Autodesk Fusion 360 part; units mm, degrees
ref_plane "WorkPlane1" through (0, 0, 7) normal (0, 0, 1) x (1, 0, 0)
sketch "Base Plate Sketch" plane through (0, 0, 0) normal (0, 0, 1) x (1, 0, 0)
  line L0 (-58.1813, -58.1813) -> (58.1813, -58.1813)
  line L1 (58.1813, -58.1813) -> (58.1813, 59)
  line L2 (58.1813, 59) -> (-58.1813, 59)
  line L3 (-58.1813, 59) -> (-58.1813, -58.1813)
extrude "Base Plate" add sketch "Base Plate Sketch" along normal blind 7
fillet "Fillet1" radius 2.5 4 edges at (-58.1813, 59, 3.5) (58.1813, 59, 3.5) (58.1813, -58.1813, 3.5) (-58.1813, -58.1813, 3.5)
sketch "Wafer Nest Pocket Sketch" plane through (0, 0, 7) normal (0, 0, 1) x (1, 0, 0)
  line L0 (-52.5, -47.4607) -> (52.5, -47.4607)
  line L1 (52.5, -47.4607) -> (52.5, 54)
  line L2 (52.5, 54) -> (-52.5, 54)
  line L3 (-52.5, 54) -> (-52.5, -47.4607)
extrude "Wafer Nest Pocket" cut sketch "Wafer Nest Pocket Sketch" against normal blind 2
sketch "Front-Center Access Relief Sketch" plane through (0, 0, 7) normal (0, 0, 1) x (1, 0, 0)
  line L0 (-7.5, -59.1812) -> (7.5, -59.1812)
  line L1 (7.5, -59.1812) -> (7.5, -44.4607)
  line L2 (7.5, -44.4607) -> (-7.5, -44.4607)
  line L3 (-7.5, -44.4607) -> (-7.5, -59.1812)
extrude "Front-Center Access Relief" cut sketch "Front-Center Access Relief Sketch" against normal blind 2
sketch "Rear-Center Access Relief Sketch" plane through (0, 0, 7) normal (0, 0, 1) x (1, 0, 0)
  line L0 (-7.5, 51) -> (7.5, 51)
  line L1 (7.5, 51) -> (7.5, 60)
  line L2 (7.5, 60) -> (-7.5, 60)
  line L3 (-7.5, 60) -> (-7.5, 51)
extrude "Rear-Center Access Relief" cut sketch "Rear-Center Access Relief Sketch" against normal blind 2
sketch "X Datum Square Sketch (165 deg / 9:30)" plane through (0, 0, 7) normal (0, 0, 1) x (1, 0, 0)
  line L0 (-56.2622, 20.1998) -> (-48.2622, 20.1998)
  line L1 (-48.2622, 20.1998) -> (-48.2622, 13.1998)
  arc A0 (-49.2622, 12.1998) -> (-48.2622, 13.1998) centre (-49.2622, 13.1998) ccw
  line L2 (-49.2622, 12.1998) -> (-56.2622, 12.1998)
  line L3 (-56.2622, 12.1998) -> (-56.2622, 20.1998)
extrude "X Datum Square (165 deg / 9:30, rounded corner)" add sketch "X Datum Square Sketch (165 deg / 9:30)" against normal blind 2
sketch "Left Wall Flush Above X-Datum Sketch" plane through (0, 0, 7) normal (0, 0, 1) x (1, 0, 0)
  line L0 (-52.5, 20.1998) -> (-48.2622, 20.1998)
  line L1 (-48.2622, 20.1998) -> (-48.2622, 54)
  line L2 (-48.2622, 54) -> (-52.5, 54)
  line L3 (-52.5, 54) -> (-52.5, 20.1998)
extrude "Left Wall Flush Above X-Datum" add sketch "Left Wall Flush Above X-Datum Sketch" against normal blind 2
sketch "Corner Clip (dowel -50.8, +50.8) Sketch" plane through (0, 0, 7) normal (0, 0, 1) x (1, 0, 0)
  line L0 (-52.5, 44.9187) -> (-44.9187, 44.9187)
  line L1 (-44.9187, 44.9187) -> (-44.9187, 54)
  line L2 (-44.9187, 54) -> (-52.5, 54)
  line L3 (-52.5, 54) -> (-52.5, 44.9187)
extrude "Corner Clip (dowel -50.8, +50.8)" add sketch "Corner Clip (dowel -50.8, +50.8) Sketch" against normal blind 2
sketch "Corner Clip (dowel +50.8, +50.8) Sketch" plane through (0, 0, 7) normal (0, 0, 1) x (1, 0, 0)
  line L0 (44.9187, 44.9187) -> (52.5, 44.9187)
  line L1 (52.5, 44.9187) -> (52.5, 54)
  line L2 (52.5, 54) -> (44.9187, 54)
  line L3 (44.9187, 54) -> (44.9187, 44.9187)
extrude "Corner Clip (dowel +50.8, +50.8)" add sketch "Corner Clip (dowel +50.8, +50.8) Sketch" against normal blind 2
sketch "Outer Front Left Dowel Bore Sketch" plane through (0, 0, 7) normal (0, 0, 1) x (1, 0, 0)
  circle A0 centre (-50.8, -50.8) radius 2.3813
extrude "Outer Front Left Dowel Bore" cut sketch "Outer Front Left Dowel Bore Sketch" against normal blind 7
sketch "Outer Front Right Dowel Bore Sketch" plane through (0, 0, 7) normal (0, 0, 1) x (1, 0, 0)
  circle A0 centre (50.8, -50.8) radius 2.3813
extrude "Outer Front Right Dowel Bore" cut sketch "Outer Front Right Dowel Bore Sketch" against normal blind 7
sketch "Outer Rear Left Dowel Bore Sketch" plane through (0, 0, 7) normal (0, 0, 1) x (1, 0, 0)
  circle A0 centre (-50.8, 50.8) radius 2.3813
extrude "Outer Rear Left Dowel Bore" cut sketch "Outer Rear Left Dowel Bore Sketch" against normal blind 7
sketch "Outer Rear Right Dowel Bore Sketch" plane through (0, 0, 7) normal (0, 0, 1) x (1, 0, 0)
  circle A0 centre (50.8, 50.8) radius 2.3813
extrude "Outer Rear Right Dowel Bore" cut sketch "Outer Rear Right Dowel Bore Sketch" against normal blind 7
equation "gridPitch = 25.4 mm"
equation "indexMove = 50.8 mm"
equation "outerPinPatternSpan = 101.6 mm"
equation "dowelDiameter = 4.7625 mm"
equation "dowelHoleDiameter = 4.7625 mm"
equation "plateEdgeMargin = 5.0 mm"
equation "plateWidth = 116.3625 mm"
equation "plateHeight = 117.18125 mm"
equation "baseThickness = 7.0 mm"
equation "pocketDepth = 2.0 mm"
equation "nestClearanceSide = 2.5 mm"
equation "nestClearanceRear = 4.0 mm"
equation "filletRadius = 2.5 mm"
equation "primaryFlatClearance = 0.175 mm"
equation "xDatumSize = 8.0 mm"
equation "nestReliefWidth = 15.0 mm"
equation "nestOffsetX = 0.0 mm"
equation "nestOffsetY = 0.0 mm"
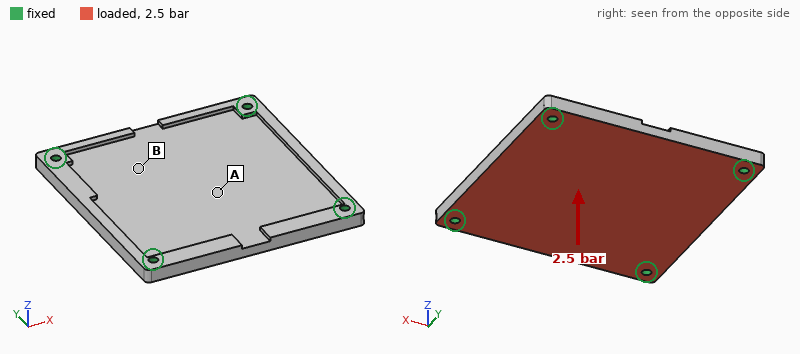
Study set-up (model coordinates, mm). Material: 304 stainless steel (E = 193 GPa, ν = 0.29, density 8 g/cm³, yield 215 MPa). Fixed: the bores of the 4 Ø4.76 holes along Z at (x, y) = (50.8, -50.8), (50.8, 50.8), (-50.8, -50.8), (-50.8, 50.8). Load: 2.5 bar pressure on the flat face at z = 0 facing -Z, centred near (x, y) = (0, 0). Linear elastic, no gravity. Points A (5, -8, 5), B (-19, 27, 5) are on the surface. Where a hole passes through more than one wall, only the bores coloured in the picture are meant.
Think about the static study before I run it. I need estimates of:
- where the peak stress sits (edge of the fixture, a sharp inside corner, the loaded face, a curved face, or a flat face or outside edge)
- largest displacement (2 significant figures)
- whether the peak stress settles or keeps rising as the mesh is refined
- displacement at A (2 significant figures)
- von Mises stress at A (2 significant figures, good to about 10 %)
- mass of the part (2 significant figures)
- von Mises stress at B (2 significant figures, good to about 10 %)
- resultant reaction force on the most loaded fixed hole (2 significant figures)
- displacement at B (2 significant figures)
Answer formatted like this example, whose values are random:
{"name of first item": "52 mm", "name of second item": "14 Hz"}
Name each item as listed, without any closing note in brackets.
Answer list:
{"where the peak stress sits": "edge of the fixture", "largest displacement": "77 µm", "whether the peak stress settles or keeps rising as the mesh is refined": "keeps rising", "displacement at A": "75 µm", "von Mises stress at A": "28 MPa", "mass of the part": "590 g", "von Mises stress at B": "18 MPa", "resultant reaction force on the most loaded fixed hole": "990 N", "displacement at B": "53 µm"}
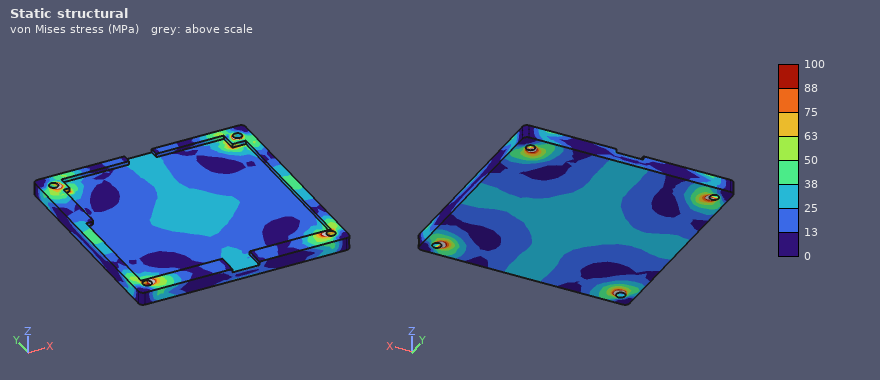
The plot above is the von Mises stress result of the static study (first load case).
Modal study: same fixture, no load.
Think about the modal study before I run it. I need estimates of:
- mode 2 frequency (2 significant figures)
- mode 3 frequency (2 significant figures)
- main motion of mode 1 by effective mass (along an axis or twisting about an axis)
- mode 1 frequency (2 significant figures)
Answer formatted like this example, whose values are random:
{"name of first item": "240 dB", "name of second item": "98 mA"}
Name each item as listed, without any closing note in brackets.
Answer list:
{"mode 2 frequency": "3000 Hz", "mode 3 frequency": "3100 Hz", "main motion of mode 1 by effective mass": "along Z", "mode 1 frequency": "1800 Hz"}
